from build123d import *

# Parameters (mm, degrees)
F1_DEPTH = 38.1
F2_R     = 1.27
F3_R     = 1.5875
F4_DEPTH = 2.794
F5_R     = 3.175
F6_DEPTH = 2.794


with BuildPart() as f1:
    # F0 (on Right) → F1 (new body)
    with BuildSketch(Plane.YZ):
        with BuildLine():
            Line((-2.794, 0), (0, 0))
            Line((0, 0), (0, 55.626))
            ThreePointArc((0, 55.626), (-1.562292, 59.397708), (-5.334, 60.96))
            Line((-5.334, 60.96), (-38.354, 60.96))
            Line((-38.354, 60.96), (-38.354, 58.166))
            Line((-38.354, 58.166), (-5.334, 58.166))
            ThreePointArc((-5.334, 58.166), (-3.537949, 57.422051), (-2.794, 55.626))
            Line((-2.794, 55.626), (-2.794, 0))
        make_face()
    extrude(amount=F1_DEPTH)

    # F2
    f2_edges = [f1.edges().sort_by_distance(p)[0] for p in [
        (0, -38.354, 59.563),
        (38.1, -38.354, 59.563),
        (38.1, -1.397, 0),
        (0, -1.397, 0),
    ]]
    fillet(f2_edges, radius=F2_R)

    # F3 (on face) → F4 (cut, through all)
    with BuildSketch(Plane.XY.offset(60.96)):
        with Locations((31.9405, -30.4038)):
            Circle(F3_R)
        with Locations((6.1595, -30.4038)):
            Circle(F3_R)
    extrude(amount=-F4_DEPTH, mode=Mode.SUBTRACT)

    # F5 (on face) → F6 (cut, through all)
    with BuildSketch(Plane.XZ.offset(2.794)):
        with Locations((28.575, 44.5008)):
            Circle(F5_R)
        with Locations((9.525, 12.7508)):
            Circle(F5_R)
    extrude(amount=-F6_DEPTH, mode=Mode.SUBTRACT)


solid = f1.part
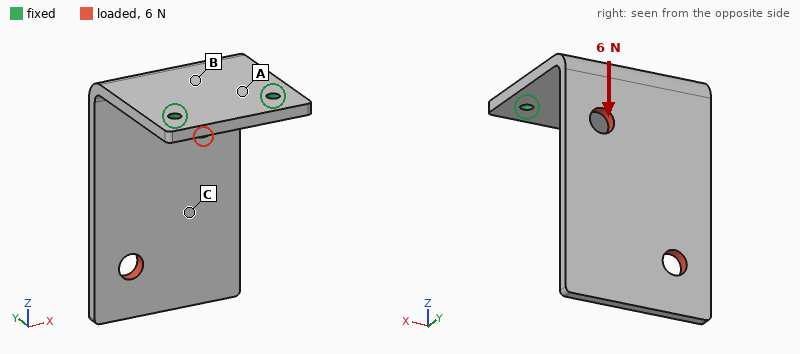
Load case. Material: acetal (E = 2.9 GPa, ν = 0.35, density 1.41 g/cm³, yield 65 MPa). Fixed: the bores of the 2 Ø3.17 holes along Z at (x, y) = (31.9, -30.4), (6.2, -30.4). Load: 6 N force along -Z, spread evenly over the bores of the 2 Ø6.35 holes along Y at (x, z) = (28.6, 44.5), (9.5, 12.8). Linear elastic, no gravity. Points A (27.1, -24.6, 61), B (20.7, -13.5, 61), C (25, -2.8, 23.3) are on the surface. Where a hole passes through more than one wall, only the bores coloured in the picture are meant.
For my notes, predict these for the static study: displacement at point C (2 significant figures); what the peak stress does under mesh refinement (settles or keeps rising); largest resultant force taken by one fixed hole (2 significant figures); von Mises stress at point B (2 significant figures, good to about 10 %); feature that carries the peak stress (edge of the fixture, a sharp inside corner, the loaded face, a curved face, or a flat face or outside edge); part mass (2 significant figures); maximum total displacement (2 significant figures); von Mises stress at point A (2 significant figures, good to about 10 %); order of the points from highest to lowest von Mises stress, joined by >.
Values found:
0.51 mm
keeps rising
3.0 N
1.3 MPa
edge of the fixture
14 g
0.79 mm
2.4 MPa
A > B > C
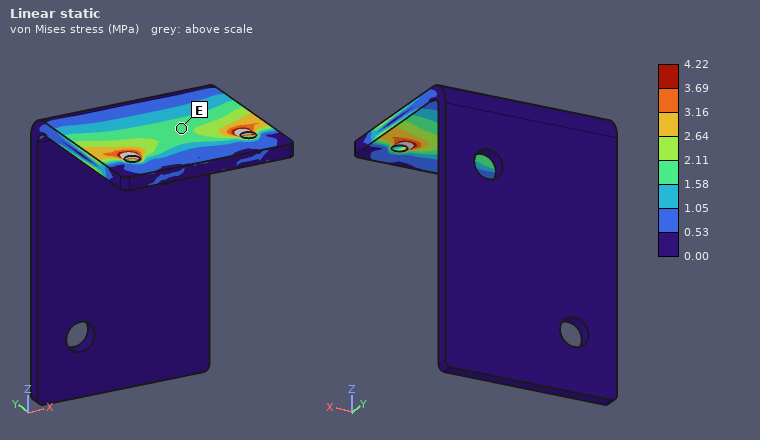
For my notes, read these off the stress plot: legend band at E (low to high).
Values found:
1.58 to 2.11 MPa
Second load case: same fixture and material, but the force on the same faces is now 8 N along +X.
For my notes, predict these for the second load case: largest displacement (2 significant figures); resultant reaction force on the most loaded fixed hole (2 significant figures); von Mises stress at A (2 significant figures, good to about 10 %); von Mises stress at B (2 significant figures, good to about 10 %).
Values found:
0.86 mm
13 N
2.4 MPa
2.9 MPa
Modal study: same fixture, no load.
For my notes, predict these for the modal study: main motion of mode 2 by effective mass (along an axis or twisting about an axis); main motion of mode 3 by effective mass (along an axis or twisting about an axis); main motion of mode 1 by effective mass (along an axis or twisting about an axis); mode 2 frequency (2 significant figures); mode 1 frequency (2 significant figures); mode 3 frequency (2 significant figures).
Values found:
along X
along Z
along Y
200 Hz
110 Hz
370 Hz
